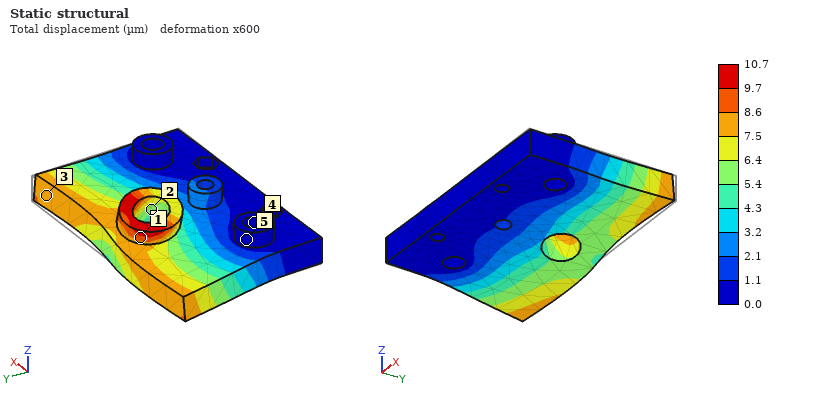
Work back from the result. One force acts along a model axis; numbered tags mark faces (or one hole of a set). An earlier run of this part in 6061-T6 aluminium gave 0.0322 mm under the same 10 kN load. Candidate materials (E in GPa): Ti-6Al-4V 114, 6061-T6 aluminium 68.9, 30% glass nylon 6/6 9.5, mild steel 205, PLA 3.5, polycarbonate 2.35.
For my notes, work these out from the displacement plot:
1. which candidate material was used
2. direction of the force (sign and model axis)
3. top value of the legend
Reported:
mild steel
-X
10.7 µm
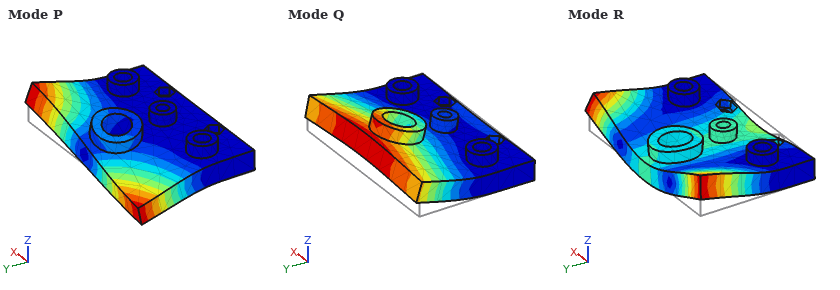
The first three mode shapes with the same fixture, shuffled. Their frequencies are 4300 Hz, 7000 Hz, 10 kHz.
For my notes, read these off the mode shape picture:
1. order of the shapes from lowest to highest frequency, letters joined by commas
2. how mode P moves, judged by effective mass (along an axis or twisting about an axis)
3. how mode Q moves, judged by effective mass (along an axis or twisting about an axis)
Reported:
Q, P, R
twisting about Y
along Z
